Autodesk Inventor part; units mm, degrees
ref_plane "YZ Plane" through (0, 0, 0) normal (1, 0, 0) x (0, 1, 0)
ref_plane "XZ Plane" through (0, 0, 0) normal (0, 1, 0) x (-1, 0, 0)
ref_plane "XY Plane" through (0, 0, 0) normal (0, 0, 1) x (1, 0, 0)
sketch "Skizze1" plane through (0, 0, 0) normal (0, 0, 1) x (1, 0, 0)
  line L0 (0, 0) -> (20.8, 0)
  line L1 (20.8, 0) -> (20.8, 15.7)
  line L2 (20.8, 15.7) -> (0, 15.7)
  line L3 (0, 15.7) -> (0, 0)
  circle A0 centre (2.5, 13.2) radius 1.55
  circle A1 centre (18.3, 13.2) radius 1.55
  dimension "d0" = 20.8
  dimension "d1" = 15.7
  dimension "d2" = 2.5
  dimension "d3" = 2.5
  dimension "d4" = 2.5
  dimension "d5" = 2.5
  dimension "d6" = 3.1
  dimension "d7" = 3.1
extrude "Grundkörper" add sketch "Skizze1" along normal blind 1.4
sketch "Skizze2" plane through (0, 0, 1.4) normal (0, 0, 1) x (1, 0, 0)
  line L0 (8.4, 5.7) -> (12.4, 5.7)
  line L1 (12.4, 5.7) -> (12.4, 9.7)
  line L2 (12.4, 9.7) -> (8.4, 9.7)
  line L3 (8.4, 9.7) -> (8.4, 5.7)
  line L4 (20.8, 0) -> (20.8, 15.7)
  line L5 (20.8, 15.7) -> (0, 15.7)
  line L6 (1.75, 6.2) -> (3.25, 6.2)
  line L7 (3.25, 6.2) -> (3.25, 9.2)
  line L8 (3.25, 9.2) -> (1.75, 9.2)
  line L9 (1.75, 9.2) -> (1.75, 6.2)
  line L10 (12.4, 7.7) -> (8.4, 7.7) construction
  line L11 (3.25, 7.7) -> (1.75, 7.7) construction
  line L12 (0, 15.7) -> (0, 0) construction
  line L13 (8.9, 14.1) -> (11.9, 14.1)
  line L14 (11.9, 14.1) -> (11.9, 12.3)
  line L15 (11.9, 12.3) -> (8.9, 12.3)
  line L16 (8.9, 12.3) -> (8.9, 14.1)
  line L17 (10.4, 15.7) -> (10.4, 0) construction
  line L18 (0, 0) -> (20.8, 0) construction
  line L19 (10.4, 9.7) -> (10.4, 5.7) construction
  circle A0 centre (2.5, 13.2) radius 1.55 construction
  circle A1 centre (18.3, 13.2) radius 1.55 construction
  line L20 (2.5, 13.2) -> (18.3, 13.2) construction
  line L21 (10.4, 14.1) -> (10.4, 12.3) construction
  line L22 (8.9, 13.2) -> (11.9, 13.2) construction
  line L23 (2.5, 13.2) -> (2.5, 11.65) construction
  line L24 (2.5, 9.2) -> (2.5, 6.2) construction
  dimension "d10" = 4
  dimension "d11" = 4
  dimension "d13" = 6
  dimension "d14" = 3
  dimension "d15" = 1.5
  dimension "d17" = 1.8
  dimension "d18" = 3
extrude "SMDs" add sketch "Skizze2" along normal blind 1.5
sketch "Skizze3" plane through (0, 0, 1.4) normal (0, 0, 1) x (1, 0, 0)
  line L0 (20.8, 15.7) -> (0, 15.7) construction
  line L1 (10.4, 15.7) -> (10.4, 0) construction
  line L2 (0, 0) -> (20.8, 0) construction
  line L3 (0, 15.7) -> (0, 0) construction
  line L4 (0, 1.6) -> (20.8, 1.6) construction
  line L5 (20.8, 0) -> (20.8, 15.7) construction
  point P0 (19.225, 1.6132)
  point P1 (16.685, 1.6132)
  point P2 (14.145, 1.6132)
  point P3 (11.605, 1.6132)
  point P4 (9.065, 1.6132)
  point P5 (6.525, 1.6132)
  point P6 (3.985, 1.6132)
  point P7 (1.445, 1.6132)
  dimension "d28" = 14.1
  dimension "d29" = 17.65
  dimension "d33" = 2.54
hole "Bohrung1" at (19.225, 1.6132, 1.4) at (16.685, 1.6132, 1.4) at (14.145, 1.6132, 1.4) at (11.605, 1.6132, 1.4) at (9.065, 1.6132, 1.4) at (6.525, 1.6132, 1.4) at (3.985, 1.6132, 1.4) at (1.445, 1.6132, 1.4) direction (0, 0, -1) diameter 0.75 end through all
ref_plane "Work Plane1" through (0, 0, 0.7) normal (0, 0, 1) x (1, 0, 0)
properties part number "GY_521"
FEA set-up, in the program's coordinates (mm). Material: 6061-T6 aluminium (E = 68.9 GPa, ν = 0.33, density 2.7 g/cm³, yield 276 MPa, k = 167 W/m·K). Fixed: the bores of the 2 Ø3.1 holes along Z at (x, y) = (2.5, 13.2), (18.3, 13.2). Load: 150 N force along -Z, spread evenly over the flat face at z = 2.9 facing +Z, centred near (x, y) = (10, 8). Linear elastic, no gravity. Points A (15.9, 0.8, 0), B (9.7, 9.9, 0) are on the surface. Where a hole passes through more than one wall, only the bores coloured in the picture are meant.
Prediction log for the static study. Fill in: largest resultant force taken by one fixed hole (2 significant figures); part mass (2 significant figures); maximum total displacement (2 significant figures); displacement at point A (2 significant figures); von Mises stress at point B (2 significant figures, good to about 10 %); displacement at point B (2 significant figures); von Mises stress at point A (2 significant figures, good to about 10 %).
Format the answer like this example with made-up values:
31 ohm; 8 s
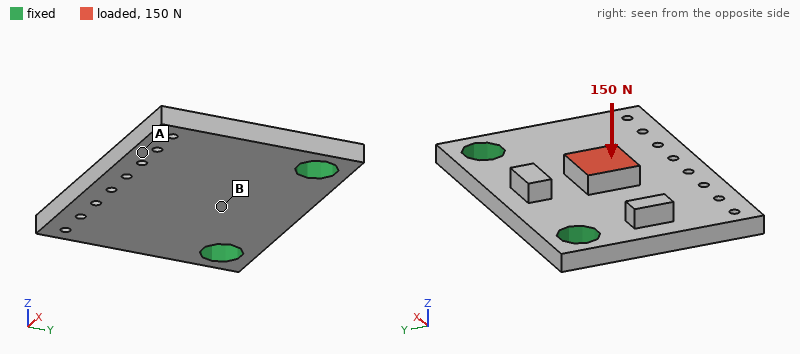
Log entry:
76 N; 1.3 g; 92 µm; 76 µm; 39 MPa; 24 µm; 16 MPa
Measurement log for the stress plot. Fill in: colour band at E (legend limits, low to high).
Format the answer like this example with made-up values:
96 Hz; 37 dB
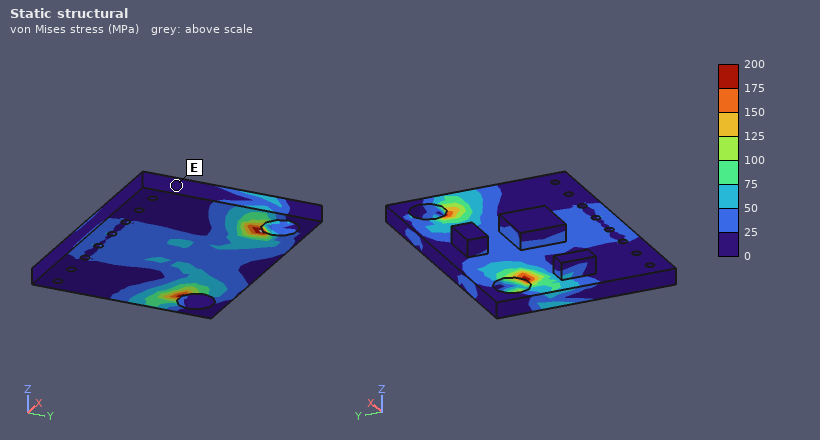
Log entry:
0 to 25 MPa
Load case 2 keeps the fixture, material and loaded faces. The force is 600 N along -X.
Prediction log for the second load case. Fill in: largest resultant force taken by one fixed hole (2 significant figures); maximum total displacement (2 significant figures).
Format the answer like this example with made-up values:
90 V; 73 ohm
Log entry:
370 N; 39 µm
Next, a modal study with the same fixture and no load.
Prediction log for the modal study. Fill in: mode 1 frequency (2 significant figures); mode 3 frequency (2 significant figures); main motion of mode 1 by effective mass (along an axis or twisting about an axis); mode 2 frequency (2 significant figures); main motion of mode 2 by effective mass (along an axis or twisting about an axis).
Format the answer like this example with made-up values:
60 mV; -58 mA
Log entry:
7200 Hz; 25 kHz; along Z; 14 kHz; twisting about Y
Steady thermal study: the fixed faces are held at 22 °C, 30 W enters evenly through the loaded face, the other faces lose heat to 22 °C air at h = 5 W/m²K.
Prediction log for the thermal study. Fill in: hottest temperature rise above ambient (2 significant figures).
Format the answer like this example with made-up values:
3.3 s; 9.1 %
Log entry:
77 K
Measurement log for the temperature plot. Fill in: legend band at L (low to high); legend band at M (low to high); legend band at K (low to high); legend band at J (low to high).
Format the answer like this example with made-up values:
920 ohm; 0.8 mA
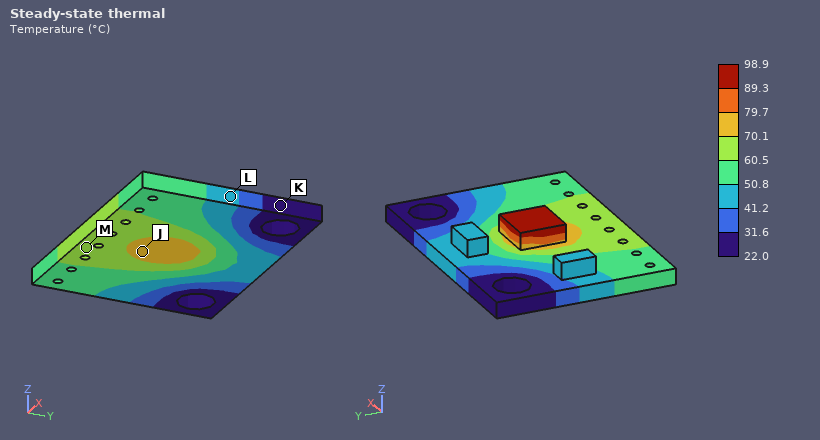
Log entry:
41.2 to 50.8 °C; 60.5 to 70.1 °C; 22.0 to 31.6 °C; 70.1 to 79.7 °C
